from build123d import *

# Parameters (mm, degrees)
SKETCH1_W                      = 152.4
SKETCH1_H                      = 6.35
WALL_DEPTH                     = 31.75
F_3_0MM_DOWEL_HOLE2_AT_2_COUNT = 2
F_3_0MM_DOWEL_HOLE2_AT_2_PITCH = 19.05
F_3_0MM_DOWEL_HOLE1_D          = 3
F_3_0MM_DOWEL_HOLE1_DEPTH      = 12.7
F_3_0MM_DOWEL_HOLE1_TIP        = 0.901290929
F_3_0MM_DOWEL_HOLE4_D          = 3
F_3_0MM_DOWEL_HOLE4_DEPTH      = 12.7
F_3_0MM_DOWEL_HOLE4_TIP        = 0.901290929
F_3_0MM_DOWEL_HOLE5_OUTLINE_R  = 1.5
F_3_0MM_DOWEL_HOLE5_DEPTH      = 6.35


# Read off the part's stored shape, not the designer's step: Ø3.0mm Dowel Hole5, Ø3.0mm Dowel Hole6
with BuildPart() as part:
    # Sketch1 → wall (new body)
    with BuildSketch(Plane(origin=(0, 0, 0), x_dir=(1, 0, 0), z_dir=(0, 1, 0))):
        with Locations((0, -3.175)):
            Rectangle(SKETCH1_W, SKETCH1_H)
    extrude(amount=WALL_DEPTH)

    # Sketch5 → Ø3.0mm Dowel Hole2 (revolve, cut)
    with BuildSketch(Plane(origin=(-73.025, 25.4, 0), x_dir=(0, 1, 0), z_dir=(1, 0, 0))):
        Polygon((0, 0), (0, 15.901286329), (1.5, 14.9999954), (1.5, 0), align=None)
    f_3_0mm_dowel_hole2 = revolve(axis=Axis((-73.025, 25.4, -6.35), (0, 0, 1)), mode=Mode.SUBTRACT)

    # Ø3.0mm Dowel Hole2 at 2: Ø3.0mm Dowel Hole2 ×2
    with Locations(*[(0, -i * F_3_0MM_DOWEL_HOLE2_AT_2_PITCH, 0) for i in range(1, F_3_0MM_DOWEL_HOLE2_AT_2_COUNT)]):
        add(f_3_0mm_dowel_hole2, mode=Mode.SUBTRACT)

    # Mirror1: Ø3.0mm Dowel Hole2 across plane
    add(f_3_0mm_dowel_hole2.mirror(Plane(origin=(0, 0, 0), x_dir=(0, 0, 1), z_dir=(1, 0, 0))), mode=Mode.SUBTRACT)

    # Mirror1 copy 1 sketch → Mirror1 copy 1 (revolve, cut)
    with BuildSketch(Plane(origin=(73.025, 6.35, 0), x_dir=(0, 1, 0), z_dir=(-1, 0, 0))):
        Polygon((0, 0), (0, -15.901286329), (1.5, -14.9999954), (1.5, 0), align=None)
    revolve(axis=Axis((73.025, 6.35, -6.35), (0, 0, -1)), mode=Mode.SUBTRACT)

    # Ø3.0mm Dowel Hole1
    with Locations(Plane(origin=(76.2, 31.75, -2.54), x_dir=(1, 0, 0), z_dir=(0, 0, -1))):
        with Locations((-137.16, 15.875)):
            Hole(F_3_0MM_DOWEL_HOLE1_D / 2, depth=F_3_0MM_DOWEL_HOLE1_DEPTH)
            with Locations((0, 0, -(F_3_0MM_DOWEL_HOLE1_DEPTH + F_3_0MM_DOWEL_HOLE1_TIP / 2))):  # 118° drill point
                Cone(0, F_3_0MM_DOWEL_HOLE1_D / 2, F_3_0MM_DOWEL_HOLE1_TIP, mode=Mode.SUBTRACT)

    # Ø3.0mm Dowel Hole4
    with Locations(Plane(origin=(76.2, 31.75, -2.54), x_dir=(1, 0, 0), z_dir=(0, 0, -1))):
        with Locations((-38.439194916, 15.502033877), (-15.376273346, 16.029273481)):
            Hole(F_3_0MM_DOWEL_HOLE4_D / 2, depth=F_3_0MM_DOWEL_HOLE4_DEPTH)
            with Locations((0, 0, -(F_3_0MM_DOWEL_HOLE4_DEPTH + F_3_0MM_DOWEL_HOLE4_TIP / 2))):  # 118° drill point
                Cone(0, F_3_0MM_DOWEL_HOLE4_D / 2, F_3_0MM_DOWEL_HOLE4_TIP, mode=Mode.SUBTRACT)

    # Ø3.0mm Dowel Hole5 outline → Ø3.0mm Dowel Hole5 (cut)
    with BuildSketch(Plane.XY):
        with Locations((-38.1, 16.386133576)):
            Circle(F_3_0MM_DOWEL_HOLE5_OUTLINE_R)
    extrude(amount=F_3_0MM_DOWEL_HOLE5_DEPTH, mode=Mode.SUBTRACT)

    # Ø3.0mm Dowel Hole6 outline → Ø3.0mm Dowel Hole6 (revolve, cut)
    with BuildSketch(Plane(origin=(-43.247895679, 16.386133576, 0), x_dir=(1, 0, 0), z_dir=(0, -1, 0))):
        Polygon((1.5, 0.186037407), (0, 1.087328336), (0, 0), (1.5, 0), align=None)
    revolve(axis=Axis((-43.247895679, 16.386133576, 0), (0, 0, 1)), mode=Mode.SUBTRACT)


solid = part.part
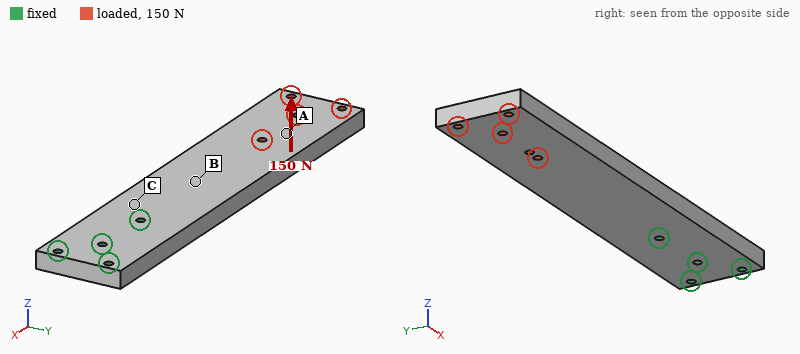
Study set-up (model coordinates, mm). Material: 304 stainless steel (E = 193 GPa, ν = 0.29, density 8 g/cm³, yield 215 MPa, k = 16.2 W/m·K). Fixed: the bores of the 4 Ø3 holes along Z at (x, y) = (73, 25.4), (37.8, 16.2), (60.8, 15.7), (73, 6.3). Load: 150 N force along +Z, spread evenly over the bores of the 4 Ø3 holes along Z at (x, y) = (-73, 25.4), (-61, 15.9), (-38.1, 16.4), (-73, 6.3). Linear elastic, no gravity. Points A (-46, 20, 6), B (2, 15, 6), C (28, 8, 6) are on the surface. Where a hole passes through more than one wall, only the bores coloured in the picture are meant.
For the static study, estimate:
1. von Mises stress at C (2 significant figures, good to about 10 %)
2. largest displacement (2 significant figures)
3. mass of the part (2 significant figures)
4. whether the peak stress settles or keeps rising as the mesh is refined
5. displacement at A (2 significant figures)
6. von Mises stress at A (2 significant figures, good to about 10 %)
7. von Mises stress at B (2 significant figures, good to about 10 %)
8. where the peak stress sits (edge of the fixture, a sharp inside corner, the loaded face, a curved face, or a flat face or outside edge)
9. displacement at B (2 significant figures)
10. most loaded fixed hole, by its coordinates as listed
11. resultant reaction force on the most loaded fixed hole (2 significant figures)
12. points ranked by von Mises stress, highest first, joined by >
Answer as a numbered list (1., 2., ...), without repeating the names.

1. 59 MPa
2. 0.49 mm
3. 240 g
4. keeps rising
5. 0.31 mm
6. 12 MPa
7. 44 MPa
8. edge of the fixture
9. 0.075 mm
10. (37.8, 16.2)
11. 490 N
12. C > B > A
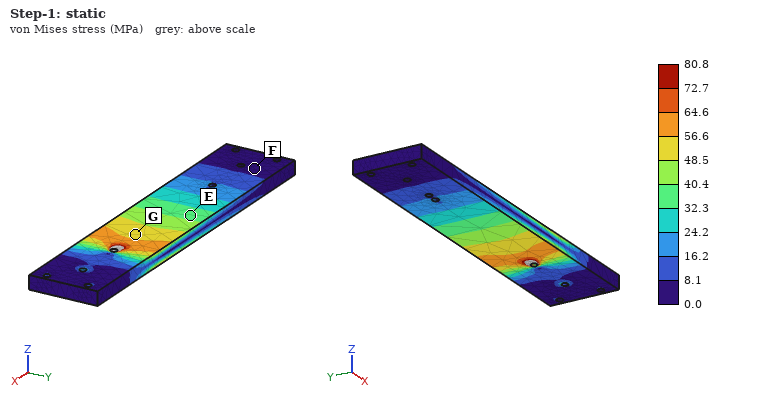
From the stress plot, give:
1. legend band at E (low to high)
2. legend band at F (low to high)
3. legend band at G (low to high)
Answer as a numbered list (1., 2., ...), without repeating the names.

1. 32.3 to 40.4 MPa
2. 0.0 to 8.1 MPa
3. 48.5 to 56.6 MPa
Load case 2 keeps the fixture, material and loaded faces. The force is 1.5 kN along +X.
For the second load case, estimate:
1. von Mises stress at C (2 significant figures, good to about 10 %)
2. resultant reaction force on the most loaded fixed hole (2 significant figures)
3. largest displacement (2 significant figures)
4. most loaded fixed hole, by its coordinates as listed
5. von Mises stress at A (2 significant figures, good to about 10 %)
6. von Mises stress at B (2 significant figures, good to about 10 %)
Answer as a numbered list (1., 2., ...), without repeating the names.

1. 7.2 MPa
2. 1.0 kN
3. 4.5 µm
4. (37.8, 16.2)
5. 5.5 MPa
6. 7.5 MPa
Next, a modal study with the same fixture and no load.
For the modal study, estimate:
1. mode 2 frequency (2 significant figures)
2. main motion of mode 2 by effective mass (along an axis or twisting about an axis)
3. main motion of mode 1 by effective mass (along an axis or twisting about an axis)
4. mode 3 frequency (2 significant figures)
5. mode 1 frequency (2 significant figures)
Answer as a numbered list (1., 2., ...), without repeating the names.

1. 1500 Hz
2. along Y
3. along Z
4. 2300 Hz
5. 380 Hz
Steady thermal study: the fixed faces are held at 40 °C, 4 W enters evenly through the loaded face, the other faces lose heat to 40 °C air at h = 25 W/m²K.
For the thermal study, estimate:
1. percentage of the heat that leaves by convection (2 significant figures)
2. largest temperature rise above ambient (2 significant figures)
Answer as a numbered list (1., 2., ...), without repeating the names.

1. 88 %
2. 38 K
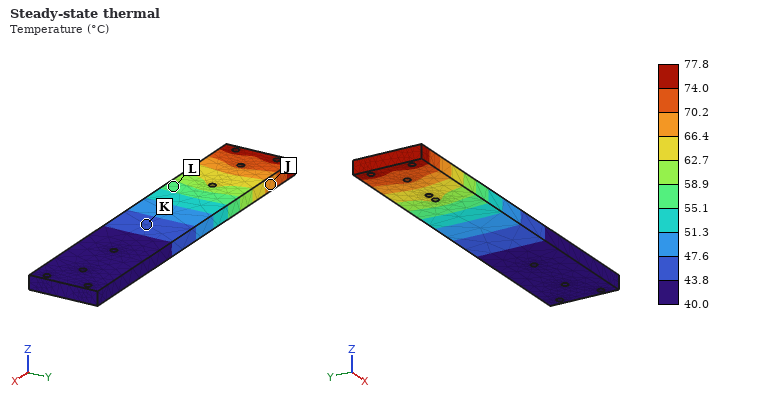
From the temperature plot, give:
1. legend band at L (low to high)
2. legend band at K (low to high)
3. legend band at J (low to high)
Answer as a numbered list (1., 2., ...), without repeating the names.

1. 55.1 to 58.9 °C
2. 43.8 to 47.6 °C
3. 66.4 to 70.2 °C
